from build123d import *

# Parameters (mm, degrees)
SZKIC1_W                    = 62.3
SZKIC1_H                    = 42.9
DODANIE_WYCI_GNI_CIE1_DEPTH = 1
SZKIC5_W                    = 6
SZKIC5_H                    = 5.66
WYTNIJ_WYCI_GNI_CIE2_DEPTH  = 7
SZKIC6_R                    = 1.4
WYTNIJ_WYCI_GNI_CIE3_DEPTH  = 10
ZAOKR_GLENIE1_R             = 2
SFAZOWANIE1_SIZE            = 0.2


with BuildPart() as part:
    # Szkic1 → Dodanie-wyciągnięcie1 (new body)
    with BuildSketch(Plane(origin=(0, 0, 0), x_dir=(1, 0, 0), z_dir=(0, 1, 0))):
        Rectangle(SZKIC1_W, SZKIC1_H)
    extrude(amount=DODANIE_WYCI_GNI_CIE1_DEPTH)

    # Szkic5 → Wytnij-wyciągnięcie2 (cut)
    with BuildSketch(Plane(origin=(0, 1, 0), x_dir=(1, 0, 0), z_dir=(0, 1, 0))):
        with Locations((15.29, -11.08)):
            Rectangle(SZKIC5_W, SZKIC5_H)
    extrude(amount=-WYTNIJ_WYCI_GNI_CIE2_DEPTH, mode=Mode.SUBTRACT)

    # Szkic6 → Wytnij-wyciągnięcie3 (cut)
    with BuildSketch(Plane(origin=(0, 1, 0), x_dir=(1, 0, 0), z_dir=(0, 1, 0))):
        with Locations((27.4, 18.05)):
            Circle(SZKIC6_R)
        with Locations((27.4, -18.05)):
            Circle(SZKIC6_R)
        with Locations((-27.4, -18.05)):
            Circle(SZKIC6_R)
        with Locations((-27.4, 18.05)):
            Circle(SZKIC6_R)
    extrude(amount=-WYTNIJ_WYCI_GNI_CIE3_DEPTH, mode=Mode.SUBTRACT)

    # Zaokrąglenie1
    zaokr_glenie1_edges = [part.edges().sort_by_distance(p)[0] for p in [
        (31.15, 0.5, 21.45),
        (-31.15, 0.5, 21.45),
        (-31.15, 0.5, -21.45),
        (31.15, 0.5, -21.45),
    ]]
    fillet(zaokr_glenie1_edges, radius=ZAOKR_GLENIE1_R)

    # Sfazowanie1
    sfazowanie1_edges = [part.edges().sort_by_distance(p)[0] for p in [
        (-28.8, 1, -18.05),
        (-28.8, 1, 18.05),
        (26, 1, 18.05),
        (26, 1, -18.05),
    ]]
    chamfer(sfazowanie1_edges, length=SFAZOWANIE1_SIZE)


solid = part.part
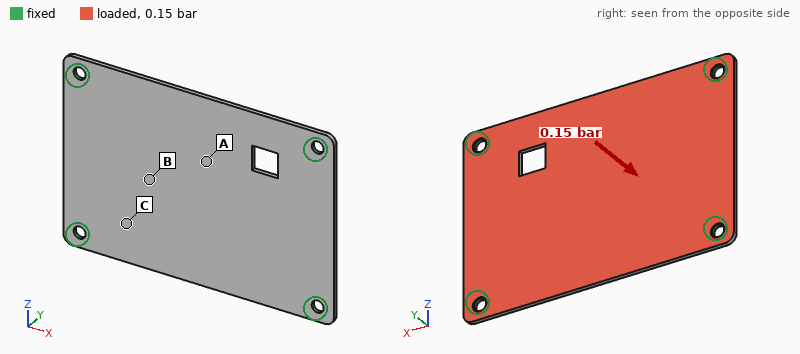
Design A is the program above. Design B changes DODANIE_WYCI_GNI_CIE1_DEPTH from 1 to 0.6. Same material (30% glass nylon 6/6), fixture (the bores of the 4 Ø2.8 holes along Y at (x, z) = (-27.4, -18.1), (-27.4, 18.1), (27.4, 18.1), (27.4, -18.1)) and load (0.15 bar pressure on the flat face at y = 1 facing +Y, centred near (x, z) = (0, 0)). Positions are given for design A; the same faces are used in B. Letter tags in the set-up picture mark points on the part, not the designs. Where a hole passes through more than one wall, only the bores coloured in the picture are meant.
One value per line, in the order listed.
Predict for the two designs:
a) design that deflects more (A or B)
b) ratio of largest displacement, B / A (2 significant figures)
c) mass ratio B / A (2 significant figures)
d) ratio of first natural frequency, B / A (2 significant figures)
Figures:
B
4.6
0.60
0.60
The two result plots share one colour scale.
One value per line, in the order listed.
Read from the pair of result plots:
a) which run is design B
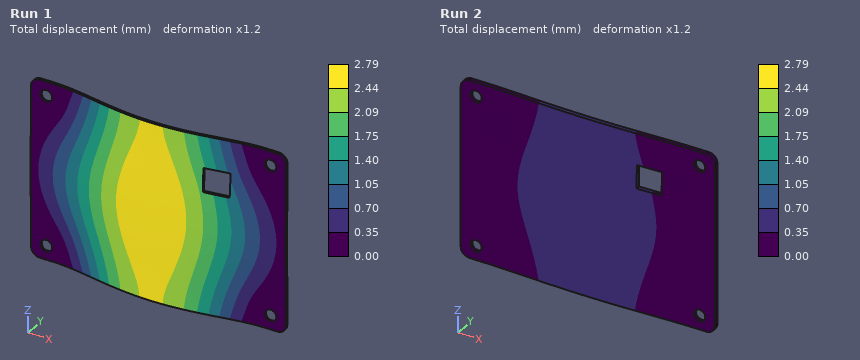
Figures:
Run 1
